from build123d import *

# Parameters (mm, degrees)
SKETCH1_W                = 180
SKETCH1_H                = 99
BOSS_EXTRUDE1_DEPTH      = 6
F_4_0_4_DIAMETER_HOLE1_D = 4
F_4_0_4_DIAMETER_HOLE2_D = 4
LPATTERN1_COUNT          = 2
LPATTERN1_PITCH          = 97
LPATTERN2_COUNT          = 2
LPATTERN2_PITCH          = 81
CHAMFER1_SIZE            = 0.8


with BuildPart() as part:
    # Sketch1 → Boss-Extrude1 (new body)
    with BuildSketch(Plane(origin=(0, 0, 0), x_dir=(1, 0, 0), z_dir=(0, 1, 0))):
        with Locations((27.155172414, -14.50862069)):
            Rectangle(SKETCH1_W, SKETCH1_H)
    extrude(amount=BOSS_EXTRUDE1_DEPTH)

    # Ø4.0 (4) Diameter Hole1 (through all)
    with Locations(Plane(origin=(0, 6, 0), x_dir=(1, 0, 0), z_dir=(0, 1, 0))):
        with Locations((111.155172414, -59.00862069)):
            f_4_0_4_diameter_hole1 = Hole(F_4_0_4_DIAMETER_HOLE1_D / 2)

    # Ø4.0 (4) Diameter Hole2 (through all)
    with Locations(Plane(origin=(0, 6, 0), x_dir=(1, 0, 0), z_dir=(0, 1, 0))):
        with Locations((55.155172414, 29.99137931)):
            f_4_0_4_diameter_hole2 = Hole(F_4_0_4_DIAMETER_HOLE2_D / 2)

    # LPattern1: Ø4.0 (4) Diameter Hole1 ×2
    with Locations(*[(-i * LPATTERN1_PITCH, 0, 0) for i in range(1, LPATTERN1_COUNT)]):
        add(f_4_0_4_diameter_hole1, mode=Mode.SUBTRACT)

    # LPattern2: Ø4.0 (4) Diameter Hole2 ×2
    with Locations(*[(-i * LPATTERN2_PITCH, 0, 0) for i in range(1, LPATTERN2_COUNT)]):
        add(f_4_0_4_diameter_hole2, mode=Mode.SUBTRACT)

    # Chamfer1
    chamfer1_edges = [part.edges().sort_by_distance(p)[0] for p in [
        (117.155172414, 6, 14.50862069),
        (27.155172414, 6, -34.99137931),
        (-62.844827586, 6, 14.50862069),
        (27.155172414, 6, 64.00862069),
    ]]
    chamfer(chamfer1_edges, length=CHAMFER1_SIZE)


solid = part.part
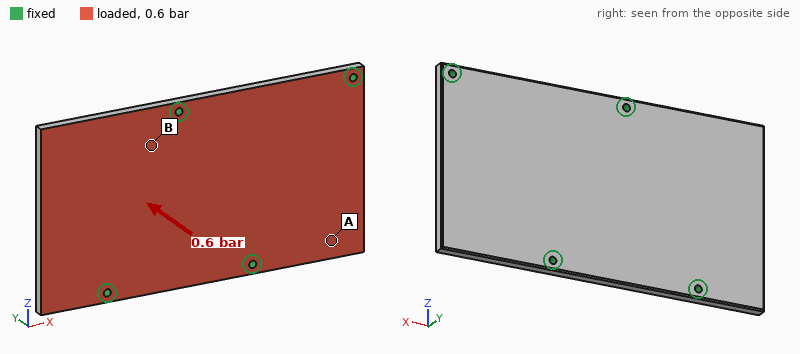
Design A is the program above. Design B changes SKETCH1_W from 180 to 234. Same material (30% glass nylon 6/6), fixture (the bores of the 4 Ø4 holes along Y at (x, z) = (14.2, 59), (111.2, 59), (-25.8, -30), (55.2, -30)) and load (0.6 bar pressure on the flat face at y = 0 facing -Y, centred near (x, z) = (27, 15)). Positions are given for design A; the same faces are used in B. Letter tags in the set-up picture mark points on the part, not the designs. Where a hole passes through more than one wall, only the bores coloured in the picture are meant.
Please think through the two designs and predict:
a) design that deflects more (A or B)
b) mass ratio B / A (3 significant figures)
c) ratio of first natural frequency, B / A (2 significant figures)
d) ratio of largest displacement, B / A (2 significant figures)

B
1.30
0.57
3.2
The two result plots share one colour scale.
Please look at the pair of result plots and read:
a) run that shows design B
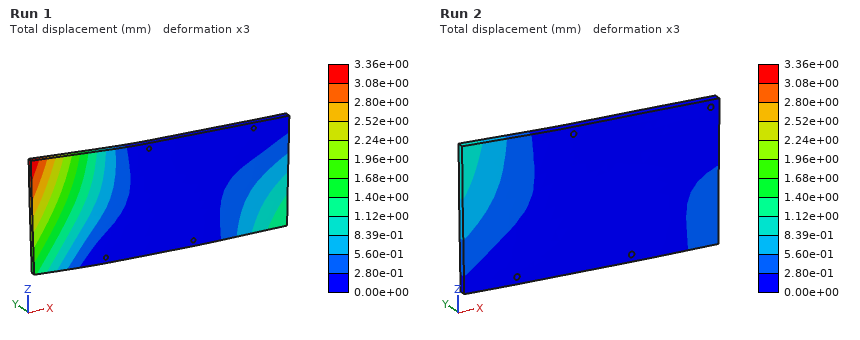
Run 1
